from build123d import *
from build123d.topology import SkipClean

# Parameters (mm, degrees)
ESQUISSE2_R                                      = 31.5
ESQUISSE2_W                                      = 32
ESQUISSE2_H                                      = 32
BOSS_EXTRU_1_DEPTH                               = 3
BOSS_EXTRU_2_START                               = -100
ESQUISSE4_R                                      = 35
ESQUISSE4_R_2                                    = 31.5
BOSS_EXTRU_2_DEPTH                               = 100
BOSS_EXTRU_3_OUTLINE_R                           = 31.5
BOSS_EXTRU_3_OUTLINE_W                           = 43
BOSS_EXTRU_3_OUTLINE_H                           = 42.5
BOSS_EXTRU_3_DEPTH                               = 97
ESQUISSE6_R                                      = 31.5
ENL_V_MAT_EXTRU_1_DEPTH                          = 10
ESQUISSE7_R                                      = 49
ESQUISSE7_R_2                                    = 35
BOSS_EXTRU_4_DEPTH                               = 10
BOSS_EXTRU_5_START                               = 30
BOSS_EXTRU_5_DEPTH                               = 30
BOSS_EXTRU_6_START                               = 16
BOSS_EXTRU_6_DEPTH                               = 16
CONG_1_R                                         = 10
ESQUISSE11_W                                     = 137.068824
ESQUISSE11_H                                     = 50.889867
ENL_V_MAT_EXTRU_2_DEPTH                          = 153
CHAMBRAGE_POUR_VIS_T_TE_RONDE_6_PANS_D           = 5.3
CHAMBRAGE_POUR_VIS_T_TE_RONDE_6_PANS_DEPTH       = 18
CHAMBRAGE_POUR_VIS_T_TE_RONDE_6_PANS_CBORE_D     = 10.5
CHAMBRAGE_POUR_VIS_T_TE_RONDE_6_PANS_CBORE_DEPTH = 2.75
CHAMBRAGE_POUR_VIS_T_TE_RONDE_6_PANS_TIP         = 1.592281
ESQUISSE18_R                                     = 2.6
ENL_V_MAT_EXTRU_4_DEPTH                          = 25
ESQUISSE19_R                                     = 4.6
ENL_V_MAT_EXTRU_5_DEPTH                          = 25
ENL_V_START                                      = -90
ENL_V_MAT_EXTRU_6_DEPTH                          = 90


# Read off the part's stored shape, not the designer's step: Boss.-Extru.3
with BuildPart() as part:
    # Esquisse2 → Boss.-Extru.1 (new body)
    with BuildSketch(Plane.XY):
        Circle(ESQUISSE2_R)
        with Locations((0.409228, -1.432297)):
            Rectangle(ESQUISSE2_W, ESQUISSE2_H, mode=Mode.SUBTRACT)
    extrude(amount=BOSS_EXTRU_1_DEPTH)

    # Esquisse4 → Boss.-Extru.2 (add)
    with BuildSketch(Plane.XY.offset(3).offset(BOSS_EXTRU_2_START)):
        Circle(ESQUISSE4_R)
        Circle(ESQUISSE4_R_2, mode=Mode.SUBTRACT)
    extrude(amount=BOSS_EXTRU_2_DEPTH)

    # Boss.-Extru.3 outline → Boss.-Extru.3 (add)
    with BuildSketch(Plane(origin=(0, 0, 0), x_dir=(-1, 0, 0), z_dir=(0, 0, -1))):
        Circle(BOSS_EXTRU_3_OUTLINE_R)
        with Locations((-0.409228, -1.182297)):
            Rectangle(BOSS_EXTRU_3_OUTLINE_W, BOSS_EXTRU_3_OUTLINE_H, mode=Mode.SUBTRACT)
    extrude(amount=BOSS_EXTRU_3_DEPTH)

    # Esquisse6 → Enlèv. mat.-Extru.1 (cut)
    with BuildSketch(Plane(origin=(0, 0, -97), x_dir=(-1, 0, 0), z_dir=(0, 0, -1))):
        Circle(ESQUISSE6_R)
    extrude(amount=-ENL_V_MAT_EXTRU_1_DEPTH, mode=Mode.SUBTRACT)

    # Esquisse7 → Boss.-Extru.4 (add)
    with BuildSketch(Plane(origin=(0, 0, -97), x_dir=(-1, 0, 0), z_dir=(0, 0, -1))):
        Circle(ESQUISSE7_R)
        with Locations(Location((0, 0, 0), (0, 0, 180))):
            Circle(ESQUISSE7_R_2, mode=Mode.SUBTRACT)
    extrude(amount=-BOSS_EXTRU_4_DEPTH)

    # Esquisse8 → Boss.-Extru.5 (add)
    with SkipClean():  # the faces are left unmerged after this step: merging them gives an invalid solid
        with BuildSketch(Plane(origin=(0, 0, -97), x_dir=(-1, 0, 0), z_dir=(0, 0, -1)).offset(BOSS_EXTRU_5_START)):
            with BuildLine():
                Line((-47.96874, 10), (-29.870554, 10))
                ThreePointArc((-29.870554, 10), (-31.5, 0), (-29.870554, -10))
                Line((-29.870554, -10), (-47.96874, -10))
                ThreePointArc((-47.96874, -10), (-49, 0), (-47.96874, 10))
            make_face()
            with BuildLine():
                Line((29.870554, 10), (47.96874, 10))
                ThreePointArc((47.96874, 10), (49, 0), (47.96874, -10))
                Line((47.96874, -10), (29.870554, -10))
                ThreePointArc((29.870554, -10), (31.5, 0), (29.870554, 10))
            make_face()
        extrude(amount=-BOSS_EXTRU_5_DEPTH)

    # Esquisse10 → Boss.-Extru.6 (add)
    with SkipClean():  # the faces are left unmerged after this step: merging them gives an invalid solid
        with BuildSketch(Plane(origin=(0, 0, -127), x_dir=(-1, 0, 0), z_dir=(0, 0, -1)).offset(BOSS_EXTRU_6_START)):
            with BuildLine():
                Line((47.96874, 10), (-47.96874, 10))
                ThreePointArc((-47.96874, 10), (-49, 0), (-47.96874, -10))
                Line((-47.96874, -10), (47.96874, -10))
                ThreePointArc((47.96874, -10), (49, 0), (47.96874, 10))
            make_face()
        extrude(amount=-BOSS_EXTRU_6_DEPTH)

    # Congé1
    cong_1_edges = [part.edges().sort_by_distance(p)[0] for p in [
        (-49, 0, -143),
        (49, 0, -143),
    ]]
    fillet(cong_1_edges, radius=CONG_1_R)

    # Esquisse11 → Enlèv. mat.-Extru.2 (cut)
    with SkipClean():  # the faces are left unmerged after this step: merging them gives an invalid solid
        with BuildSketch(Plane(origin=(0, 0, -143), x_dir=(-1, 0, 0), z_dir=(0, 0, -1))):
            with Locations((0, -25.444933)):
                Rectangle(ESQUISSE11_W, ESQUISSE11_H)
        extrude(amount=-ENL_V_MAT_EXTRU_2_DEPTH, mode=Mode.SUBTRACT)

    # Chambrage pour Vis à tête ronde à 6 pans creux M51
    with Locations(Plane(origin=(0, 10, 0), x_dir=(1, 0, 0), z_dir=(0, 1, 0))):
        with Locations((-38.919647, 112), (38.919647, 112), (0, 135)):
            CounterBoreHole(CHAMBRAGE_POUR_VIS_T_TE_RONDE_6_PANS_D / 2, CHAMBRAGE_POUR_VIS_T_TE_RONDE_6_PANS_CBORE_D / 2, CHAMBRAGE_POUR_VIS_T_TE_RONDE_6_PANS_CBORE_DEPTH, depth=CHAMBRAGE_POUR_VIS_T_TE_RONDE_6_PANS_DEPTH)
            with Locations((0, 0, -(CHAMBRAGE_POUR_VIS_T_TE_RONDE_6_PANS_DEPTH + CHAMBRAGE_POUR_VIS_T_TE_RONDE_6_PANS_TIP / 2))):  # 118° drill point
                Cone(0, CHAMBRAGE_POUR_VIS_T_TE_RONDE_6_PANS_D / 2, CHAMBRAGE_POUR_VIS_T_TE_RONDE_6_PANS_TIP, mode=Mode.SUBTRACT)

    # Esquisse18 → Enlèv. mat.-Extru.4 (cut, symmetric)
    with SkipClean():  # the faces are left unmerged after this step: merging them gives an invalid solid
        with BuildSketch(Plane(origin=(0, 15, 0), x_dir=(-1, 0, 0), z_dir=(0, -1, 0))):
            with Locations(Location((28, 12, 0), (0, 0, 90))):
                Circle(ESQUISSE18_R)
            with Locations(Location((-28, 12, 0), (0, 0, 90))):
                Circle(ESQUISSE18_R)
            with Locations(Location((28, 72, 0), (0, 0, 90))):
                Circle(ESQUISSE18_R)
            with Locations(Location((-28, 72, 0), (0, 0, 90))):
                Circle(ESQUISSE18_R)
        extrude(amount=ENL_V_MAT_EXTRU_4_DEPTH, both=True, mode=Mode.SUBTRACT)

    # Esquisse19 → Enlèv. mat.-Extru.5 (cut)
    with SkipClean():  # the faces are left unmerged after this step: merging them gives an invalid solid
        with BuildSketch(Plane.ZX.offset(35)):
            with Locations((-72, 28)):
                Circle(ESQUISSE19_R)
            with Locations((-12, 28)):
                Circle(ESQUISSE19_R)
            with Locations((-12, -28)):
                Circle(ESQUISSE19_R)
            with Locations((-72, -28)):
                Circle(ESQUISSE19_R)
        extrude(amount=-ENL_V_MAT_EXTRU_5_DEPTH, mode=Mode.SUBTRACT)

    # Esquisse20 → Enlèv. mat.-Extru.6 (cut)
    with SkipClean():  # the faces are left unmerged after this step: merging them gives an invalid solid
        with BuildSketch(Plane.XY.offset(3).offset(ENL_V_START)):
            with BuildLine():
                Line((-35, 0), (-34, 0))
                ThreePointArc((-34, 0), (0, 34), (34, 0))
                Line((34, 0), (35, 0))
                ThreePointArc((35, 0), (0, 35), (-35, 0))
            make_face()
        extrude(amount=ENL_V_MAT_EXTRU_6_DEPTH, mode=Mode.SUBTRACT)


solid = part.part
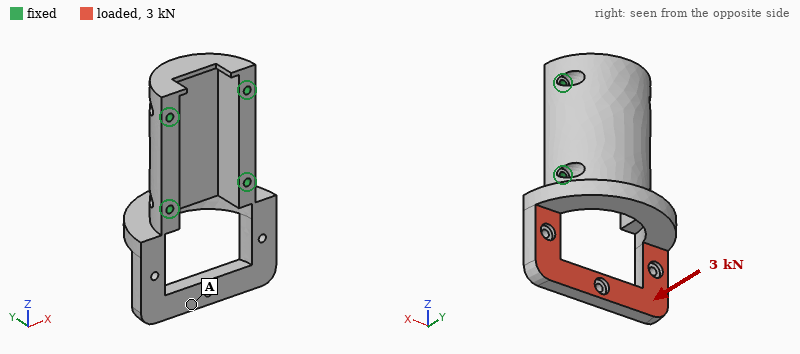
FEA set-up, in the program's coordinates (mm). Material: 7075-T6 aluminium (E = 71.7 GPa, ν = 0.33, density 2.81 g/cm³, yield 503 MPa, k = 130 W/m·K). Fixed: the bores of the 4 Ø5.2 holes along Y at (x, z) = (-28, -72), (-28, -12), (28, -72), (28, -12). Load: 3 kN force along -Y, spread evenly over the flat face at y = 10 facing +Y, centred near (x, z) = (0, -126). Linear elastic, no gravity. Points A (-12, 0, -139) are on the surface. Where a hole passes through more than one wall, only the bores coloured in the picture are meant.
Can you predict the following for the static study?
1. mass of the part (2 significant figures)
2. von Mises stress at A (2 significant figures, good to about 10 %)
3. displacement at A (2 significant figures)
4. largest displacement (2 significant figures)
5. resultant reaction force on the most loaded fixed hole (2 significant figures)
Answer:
370 g
28 MPa
0.68 mm
0.75 mm
3.0 kN
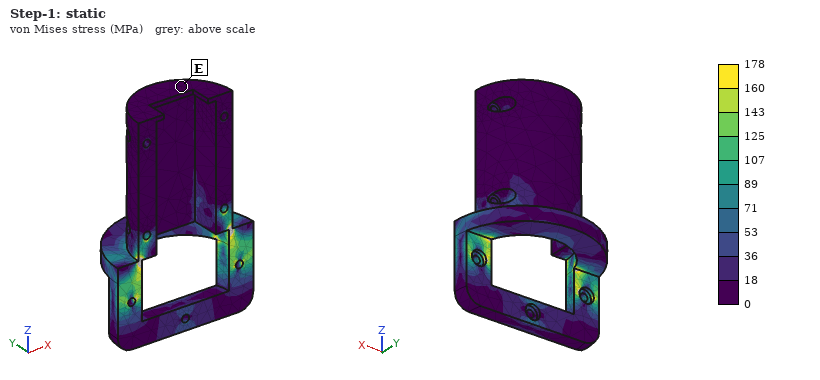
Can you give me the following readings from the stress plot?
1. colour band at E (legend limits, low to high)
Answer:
0 to 18 MPa
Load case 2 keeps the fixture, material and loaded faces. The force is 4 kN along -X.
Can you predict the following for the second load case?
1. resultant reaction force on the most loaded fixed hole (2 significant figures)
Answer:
3.3 kN
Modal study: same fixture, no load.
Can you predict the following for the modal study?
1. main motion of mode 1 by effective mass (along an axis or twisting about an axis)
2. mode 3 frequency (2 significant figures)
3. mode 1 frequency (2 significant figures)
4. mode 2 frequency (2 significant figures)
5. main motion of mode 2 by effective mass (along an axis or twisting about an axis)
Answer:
along Y
2800 Hz
1400 Hz
1800 Hz
along X
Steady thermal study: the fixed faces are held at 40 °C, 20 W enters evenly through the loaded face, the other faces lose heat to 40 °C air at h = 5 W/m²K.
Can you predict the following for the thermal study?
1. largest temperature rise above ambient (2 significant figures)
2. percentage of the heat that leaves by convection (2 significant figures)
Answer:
28 K
5.6 %
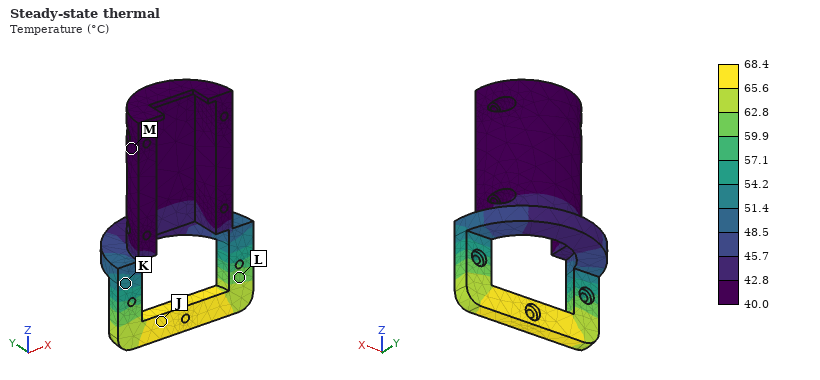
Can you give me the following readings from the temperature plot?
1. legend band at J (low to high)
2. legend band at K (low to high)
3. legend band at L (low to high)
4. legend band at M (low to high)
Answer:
65.6 to 68.4 °C
51.4 to 54.2 °C
59.9 to 62.8 °C
40.0 to 42.8 °C
